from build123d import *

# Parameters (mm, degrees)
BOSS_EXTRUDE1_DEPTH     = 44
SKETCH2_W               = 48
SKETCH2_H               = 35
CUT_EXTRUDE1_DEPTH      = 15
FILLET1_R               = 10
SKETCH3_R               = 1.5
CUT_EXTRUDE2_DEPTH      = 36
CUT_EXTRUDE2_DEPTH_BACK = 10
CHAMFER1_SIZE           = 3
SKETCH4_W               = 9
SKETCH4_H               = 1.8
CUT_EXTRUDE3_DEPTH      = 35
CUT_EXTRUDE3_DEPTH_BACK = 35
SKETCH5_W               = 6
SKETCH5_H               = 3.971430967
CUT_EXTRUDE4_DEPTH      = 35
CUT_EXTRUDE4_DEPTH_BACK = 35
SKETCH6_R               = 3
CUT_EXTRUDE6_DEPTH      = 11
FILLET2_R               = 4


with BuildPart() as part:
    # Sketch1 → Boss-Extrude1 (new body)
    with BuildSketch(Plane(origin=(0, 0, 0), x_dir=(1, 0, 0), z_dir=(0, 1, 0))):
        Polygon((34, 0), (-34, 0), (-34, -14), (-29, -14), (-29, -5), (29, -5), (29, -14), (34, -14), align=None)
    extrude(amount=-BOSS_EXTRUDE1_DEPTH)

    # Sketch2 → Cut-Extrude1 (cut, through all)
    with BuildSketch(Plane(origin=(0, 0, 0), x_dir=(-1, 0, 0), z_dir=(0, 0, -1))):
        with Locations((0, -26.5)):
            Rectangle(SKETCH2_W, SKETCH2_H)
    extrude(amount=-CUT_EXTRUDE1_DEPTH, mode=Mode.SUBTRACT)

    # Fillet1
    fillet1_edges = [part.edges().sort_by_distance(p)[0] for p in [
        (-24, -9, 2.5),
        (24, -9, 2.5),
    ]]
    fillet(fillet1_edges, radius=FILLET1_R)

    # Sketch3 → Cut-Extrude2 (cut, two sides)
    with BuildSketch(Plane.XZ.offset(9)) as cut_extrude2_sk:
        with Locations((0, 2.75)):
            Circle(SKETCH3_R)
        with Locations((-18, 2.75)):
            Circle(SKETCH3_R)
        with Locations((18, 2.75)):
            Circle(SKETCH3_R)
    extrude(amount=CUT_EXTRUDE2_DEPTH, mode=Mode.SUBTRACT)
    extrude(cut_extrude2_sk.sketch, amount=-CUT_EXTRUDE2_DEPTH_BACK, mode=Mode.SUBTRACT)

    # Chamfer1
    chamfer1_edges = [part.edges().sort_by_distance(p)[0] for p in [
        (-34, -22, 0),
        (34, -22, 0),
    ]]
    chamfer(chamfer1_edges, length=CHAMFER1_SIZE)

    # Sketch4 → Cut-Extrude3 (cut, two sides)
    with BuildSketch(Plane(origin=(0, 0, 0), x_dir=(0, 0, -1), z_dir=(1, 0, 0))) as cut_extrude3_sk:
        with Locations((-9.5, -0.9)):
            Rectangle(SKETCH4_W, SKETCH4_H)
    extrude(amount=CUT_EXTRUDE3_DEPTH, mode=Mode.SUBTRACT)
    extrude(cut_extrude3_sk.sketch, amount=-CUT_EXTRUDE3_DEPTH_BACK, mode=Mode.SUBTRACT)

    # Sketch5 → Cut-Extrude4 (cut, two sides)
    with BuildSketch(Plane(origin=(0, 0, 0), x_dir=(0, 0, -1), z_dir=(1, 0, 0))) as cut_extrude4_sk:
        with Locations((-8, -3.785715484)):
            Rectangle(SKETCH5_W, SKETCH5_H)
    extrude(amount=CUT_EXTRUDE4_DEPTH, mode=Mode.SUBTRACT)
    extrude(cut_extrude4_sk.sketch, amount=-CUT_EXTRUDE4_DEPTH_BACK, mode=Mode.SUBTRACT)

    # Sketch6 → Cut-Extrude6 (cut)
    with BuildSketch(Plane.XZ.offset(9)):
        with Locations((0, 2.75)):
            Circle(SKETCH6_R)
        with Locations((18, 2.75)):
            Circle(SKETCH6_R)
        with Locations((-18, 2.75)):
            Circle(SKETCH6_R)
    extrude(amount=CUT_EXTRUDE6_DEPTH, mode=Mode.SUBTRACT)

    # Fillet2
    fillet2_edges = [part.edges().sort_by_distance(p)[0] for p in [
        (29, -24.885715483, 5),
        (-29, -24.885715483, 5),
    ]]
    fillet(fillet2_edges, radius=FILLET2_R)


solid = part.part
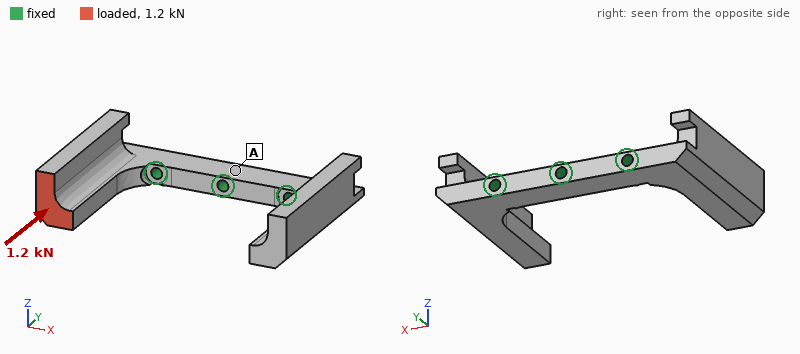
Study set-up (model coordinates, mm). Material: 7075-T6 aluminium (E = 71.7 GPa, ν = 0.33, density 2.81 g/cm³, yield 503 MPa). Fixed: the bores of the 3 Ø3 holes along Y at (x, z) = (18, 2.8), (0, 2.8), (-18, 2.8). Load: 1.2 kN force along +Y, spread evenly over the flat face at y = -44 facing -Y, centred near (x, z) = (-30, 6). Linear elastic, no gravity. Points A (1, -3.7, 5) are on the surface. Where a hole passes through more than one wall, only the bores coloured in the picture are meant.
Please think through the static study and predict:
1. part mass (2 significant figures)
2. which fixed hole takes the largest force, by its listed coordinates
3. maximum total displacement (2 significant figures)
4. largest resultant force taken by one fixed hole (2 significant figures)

28 g
(-18, 2.8)
0.24 mm
1.2 kN
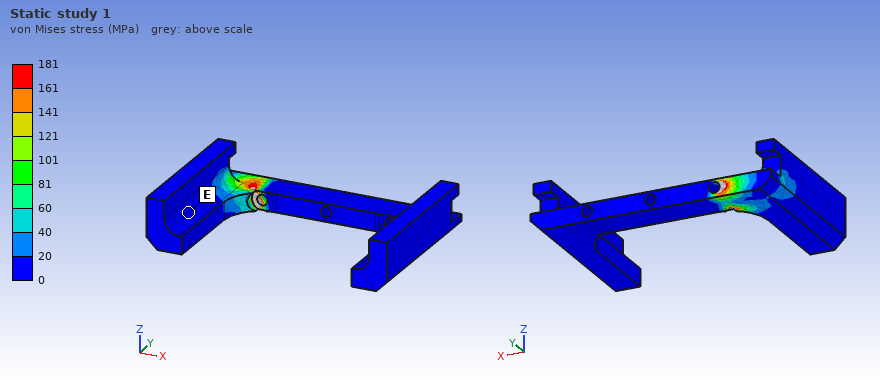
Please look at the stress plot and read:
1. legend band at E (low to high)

0 to 20 MPa
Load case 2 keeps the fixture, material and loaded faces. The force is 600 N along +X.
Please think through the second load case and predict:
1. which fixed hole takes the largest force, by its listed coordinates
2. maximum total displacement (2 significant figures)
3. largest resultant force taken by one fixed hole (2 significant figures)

(-18, 2.8)
0.58 mm
600 N
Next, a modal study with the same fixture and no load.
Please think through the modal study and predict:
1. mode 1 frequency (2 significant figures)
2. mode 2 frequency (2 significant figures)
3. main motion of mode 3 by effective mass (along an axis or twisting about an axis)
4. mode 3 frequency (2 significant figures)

1900 Hz
1900 Hz
along X
3100 Hz
